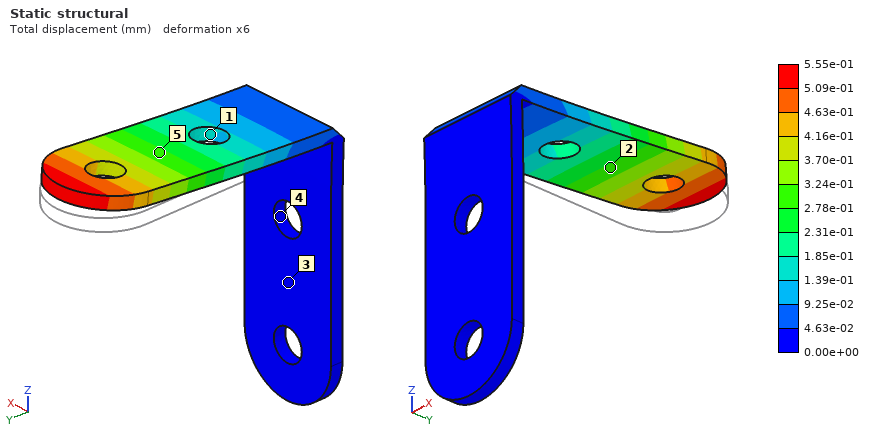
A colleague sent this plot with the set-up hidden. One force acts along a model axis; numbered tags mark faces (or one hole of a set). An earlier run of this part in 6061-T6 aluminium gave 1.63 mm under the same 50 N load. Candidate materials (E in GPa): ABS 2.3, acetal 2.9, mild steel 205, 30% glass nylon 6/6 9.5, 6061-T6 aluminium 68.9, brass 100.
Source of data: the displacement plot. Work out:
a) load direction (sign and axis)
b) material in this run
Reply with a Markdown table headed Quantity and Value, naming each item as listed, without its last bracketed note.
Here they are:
| Quantity | Value |
|---|---|
| load direction | +Z |
| material in this run | mild steel |
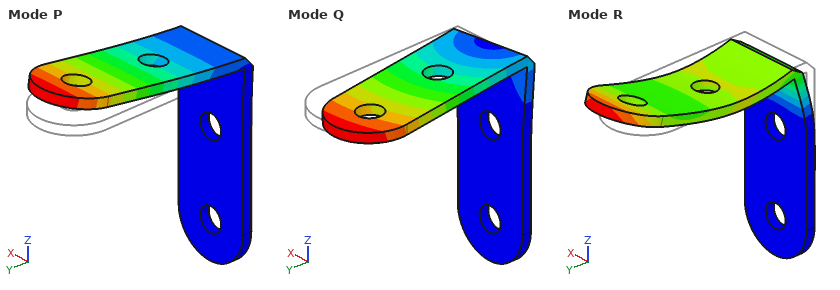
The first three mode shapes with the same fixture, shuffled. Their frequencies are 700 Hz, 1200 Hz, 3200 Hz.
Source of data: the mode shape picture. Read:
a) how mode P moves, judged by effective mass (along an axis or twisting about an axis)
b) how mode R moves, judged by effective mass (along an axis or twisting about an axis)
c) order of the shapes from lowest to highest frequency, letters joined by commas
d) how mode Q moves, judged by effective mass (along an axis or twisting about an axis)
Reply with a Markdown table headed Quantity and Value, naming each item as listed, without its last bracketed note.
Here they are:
| Quantity | Value |
|---|---|
| how mode P moves, judged by effective mass | along Z |
| how mode R moves, judged by effective mass | along Y |
| order of the shapes from lowest to highest frequency, letters joined by commas | P, Q, R |
| how mode Q moves, judged by effective mass | along X |
